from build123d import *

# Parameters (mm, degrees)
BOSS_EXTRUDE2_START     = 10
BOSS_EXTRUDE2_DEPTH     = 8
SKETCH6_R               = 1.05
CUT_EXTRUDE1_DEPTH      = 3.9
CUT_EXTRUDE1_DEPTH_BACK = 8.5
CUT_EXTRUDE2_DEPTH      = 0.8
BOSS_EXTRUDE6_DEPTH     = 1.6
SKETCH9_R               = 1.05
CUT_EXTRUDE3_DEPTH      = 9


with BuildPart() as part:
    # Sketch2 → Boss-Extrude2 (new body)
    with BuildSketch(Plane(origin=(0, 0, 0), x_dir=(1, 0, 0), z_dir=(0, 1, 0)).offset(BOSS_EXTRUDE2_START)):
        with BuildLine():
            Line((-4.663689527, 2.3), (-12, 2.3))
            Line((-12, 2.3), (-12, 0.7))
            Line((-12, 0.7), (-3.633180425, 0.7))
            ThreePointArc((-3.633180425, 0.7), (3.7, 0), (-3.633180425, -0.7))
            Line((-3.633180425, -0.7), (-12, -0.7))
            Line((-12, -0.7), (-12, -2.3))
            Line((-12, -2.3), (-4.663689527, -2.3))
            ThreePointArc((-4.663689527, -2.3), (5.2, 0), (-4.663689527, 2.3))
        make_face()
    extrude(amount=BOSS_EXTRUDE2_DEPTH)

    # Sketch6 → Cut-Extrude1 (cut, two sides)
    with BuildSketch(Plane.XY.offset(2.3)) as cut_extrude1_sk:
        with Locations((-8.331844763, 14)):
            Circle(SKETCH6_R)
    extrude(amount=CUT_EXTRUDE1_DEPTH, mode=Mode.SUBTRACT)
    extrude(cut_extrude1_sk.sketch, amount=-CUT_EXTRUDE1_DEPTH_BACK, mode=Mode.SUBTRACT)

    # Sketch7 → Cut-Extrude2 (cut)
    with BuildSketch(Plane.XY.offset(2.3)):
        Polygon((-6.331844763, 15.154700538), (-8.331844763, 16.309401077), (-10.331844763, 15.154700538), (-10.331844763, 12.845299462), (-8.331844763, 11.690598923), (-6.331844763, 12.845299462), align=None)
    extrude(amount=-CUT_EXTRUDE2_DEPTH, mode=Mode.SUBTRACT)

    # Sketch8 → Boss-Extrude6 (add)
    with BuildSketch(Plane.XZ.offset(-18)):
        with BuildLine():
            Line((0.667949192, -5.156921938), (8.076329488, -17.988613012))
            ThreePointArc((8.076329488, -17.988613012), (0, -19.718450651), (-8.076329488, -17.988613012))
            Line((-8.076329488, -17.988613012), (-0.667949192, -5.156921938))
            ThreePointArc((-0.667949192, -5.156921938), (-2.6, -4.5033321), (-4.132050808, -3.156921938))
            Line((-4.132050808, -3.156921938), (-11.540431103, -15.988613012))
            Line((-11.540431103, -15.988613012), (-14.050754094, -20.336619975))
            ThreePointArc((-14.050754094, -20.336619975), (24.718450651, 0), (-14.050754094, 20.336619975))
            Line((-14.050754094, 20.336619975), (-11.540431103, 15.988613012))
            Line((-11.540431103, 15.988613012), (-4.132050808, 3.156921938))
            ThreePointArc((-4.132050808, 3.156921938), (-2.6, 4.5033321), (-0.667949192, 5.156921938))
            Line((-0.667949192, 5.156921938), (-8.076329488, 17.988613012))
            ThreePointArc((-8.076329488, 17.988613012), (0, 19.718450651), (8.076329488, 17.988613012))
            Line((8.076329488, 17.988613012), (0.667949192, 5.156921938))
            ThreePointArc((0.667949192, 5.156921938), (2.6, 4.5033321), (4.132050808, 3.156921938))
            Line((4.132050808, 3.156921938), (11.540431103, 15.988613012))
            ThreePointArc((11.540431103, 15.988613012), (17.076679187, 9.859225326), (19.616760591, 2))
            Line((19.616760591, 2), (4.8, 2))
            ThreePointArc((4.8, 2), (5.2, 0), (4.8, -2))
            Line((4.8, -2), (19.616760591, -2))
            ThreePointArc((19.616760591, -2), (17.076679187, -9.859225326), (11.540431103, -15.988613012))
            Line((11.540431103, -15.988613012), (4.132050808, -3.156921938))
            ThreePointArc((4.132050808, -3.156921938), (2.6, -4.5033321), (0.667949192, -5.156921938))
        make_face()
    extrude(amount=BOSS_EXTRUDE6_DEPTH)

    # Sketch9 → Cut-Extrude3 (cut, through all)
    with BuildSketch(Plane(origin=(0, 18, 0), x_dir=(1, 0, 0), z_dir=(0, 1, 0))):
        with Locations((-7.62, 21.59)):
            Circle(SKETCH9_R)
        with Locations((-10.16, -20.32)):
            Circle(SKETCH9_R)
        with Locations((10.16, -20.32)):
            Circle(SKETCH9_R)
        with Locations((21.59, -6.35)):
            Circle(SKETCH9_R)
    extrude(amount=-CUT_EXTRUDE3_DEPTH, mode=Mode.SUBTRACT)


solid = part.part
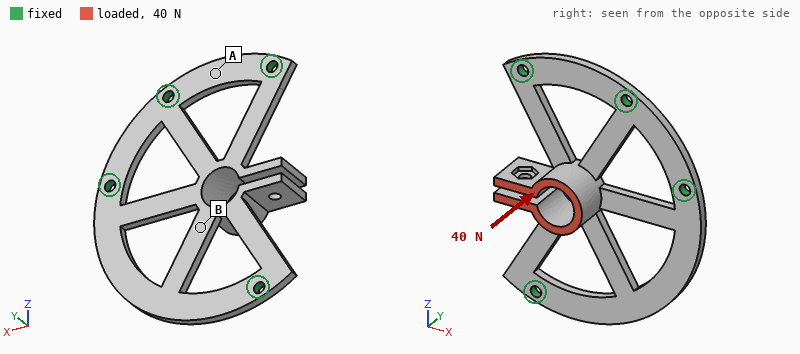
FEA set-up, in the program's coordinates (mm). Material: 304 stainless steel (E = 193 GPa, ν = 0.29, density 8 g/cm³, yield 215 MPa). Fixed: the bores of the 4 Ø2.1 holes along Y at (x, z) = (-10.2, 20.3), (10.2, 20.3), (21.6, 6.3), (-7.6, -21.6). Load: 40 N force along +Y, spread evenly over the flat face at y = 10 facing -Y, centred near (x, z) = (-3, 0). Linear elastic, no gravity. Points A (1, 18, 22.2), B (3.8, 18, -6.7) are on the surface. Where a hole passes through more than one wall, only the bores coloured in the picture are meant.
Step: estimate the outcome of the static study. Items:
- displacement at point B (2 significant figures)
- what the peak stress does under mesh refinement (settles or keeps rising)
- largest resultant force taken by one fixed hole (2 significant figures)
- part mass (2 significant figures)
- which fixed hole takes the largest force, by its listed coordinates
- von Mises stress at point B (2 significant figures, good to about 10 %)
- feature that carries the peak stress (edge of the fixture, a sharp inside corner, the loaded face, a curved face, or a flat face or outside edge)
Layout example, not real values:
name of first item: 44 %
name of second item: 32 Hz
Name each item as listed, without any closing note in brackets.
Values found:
displacement at point B: 18 µm
what the peak stress does under mesh refinement: keeps rising
largest resultant force taken by one fixed hole: 18 N
part mass: 14 g
which fixed hole takes the largest force, by its listed coordinates: (-7.6, -21.6)
von Mises stress at point B: 17 MPa
feature that carries the peak stress: edge of the fixture
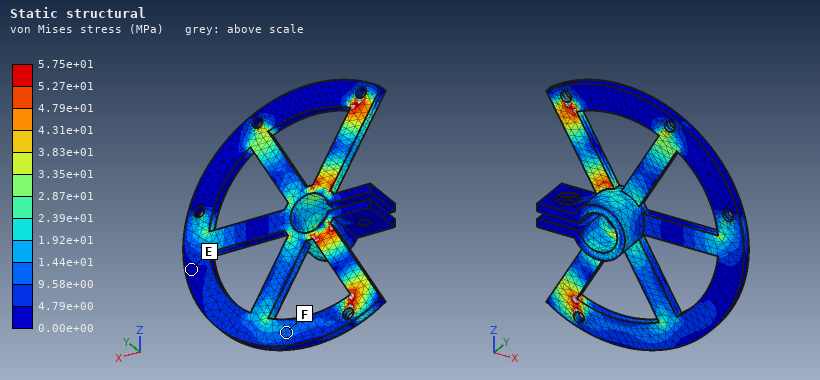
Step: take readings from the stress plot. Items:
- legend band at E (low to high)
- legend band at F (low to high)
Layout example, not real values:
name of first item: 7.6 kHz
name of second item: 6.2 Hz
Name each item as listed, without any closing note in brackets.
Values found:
legend band at E: 0.00e+00 to 4.79e+00 MPa
legend band at F: 9.58e+00 to 1.44e+01 MPa
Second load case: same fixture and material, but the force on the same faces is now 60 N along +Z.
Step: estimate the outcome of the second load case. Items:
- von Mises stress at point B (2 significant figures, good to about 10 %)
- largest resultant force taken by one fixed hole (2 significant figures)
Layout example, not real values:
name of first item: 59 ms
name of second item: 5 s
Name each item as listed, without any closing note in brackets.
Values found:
von Mises stress at point B: 29 MPa
largest resultant force taken by one fixed hole: 25 N
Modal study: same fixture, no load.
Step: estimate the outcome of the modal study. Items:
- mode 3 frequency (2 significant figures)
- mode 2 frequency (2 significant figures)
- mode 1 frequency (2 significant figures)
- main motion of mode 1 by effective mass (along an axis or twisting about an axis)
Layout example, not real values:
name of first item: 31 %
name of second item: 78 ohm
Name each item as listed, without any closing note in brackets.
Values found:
mode 3 frequency: 5600 Hz
mode 2 frequency: 3200 Hz
mode 1 frequency: 2700 Hz
main motion of mode 1 by effective mass: along Y
